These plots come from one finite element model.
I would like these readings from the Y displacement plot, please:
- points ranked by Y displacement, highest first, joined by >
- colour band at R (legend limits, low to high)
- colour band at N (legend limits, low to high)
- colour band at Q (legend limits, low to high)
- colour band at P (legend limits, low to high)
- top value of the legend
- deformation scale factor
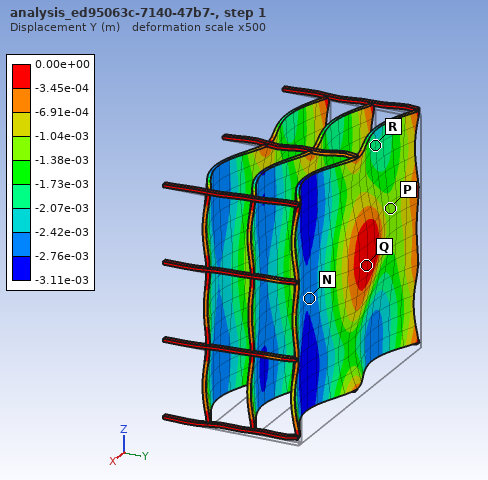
Q > P > R > N
-2.07e-03 to -1.73e-03 m
-2.76e-03 to -2.42e-03 m
-3.45e-04 to 0.00e+00 m
-1.38e-03 to -1.04e-03 m
0.00e+00 m
500
